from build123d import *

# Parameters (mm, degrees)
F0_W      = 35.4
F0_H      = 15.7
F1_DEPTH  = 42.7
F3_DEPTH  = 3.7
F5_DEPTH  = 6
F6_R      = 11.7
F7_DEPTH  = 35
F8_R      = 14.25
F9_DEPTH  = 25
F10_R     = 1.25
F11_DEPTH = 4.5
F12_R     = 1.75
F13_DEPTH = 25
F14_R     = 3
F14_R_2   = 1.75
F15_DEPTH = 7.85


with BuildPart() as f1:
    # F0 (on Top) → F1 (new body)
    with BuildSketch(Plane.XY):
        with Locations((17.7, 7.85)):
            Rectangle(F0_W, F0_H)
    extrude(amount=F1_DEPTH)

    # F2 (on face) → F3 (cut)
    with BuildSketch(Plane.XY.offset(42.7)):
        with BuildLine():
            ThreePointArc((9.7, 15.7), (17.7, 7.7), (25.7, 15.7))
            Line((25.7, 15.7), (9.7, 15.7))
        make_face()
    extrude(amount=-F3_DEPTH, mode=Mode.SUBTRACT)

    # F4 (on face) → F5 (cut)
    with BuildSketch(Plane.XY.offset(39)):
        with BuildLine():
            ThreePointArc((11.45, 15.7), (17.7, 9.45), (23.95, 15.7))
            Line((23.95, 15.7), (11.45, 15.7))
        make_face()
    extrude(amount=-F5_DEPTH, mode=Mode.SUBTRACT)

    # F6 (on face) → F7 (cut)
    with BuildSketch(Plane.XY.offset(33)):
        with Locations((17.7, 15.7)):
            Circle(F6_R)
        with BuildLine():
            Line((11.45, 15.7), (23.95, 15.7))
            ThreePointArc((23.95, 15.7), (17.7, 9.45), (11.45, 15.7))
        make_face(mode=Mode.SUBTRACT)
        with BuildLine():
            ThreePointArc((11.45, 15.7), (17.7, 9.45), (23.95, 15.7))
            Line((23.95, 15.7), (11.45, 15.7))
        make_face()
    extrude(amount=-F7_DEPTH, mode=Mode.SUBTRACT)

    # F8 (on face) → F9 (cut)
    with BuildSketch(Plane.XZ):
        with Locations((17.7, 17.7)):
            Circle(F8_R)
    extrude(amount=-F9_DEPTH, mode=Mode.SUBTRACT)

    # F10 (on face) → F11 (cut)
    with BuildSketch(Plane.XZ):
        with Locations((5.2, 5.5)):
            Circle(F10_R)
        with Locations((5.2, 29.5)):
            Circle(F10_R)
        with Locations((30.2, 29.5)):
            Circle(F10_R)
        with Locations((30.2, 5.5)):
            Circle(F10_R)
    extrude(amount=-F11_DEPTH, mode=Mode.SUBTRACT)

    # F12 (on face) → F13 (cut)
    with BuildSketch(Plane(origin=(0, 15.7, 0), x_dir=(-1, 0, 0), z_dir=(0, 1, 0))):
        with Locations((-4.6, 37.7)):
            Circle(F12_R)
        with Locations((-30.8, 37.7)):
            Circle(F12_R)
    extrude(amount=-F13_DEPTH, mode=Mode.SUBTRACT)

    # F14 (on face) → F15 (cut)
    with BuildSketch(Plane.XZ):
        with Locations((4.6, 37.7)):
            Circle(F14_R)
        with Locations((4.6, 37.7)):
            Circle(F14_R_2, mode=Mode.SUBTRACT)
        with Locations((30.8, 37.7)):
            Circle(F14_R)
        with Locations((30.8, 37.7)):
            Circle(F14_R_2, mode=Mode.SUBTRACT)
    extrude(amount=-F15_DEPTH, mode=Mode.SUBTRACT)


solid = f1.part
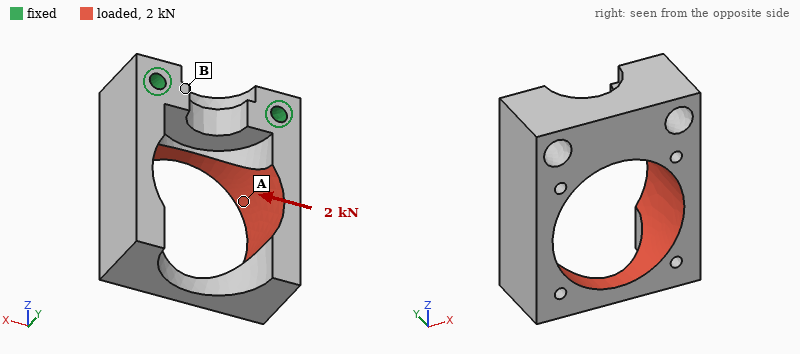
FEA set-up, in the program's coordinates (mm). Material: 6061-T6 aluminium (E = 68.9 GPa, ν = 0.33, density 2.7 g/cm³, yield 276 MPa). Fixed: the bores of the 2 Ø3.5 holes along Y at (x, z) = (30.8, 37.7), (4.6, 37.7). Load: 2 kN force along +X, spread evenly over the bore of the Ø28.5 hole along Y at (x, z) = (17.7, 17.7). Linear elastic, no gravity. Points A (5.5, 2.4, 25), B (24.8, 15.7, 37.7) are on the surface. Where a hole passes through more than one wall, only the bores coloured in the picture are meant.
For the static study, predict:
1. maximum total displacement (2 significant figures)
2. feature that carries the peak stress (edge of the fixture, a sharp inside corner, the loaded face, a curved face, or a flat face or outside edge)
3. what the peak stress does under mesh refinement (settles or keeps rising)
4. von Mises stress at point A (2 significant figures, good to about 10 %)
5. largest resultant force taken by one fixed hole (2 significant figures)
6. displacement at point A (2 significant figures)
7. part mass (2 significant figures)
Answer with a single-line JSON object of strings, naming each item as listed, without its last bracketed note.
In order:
{"maximum total displacement": "0.14 mm", "feature that carries the peak stress": "edge of the fixture", "what the peak stress does under mesh refinement": "keeps rising", "von Mises stress at point A": "74 MPa", "largest resultant force taken by one fixed hole": "1.5 kN", "displacement at point A": "0.024 mm", "part mass": "29 g"}
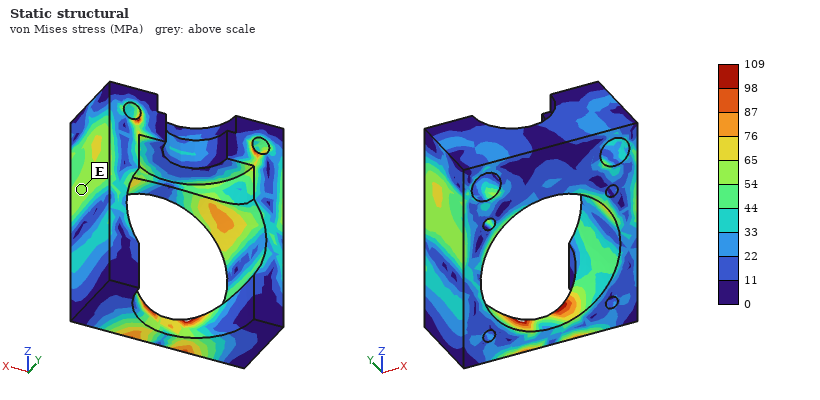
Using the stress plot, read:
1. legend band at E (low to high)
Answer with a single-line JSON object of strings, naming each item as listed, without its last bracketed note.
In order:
{"legend band at E": "54 to 65 MPa"}
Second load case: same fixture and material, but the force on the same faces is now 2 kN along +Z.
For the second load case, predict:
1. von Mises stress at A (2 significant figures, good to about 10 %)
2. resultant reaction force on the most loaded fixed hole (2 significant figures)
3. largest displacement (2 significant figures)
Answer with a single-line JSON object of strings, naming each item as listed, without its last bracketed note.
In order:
{"von Mises stress at A": "6.4 MPa", "resultant reaction force on the most loaded fixed hole": "1.0 kN", "largest displacement": "47 µm"}
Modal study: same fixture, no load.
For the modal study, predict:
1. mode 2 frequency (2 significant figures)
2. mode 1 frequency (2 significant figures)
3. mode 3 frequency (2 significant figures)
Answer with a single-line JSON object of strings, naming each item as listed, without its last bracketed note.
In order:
{"mode 2 frequency": "4800 Hz", "mode 1 frequency": "4700 Hz", "mode 3 frequency": "7800 Hz"}
